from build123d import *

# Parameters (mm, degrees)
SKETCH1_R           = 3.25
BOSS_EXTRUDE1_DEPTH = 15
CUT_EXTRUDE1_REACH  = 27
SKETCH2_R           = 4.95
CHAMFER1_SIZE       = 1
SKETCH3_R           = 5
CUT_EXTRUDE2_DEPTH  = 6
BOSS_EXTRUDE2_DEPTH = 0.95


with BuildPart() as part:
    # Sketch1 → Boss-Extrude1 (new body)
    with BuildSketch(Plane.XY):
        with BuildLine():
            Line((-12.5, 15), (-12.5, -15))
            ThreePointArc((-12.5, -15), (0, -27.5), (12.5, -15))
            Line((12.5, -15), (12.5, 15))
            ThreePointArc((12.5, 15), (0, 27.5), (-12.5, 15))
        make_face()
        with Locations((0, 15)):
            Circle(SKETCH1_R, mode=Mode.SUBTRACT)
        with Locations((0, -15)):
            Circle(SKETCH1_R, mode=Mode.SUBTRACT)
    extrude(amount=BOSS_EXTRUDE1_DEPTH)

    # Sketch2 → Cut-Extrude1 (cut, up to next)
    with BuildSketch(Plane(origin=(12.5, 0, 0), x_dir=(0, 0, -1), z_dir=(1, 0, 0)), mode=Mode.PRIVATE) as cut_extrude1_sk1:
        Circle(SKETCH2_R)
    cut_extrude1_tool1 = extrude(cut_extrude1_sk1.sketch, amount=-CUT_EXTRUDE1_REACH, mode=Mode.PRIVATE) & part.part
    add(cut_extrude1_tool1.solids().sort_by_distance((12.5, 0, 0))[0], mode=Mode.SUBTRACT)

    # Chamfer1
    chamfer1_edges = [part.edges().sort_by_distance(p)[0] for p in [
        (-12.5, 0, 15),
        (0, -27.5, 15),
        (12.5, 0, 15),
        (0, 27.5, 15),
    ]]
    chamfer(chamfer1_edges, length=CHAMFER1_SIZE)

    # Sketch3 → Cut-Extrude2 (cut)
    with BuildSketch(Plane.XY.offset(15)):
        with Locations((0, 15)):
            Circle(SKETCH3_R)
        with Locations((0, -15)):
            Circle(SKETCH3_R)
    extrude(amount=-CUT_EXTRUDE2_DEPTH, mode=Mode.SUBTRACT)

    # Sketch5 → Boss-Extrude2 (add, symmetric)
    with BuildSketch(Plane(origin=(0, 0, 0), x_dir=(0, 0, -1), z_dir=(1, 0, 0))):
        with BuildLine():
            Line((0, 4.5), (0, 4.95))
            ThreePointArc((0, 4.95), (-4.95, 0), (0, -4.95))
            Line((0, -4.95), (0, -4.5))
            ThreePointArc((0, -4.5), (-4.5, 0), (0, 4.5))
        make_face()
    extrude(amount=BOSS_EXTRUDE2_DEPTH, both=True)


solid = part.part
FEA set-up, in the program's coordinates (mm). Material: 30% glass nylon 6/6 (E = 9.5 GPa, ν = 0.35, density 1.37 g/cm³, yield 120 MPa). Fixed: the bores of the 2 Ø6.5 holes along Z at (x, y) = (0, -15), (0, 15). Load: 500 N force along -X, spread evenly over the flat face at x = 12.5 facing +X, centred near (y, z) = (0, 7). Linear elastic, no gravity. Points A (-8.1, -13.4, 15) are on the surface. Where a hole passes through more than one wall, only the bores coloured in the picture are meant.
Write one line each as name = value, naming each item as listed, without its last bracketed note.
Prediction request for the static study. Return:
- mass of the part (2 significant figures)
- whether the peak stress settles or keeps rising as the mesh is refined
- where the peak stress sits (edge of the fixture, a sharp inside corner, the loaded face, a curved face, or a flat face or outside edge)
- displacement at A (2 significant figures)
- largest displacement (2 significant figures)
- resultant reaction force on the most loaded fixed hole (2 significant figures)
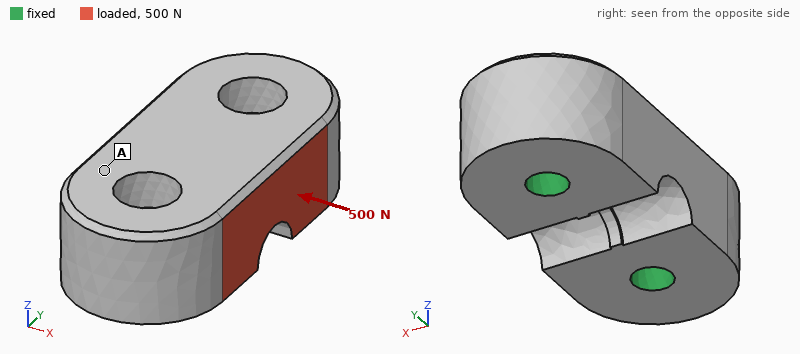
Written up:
mass of the part = 22 g
whether the peak stress settles or keeps rising as the mesh is refined = keeps rising
where the peak stress sits = edge of the fixture
displacement at A = 2.8 µm
largest displacement = 6.3 µm
resultant reaction force on the most loaded fixed hole = 250 N
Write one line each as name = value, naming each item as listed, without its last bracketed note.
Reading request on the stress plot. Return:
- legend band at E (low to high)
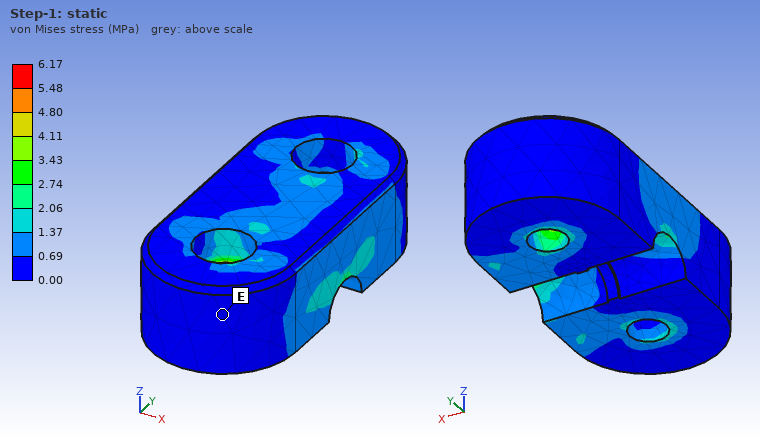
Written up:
legend band at E = 0.00 to 0.69 MPa
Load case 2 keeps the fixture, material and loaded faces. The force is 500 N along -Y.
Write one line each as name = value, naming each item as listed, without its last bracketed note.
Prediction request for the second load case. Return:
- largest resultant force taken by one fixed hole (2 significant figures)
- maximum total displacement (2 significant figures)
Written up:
largest resultant force taken by one fixed hole = 300 N
maximum total displacement = 6.2 µm
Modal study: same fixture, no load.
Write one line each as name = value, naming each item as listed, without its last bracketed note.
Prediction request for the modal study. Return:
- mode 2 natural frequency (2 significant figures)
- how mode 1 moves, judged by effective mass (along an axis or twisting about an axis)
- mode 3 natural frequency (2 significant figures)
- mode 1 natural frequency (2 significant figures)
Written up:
mode 2 natural frequency = 16 kHz
how mode 1 moves, judged by effective mass = along X
mode 3 natural frequency = 17 kHz
mode 1 natural frequency = 12 kHz
